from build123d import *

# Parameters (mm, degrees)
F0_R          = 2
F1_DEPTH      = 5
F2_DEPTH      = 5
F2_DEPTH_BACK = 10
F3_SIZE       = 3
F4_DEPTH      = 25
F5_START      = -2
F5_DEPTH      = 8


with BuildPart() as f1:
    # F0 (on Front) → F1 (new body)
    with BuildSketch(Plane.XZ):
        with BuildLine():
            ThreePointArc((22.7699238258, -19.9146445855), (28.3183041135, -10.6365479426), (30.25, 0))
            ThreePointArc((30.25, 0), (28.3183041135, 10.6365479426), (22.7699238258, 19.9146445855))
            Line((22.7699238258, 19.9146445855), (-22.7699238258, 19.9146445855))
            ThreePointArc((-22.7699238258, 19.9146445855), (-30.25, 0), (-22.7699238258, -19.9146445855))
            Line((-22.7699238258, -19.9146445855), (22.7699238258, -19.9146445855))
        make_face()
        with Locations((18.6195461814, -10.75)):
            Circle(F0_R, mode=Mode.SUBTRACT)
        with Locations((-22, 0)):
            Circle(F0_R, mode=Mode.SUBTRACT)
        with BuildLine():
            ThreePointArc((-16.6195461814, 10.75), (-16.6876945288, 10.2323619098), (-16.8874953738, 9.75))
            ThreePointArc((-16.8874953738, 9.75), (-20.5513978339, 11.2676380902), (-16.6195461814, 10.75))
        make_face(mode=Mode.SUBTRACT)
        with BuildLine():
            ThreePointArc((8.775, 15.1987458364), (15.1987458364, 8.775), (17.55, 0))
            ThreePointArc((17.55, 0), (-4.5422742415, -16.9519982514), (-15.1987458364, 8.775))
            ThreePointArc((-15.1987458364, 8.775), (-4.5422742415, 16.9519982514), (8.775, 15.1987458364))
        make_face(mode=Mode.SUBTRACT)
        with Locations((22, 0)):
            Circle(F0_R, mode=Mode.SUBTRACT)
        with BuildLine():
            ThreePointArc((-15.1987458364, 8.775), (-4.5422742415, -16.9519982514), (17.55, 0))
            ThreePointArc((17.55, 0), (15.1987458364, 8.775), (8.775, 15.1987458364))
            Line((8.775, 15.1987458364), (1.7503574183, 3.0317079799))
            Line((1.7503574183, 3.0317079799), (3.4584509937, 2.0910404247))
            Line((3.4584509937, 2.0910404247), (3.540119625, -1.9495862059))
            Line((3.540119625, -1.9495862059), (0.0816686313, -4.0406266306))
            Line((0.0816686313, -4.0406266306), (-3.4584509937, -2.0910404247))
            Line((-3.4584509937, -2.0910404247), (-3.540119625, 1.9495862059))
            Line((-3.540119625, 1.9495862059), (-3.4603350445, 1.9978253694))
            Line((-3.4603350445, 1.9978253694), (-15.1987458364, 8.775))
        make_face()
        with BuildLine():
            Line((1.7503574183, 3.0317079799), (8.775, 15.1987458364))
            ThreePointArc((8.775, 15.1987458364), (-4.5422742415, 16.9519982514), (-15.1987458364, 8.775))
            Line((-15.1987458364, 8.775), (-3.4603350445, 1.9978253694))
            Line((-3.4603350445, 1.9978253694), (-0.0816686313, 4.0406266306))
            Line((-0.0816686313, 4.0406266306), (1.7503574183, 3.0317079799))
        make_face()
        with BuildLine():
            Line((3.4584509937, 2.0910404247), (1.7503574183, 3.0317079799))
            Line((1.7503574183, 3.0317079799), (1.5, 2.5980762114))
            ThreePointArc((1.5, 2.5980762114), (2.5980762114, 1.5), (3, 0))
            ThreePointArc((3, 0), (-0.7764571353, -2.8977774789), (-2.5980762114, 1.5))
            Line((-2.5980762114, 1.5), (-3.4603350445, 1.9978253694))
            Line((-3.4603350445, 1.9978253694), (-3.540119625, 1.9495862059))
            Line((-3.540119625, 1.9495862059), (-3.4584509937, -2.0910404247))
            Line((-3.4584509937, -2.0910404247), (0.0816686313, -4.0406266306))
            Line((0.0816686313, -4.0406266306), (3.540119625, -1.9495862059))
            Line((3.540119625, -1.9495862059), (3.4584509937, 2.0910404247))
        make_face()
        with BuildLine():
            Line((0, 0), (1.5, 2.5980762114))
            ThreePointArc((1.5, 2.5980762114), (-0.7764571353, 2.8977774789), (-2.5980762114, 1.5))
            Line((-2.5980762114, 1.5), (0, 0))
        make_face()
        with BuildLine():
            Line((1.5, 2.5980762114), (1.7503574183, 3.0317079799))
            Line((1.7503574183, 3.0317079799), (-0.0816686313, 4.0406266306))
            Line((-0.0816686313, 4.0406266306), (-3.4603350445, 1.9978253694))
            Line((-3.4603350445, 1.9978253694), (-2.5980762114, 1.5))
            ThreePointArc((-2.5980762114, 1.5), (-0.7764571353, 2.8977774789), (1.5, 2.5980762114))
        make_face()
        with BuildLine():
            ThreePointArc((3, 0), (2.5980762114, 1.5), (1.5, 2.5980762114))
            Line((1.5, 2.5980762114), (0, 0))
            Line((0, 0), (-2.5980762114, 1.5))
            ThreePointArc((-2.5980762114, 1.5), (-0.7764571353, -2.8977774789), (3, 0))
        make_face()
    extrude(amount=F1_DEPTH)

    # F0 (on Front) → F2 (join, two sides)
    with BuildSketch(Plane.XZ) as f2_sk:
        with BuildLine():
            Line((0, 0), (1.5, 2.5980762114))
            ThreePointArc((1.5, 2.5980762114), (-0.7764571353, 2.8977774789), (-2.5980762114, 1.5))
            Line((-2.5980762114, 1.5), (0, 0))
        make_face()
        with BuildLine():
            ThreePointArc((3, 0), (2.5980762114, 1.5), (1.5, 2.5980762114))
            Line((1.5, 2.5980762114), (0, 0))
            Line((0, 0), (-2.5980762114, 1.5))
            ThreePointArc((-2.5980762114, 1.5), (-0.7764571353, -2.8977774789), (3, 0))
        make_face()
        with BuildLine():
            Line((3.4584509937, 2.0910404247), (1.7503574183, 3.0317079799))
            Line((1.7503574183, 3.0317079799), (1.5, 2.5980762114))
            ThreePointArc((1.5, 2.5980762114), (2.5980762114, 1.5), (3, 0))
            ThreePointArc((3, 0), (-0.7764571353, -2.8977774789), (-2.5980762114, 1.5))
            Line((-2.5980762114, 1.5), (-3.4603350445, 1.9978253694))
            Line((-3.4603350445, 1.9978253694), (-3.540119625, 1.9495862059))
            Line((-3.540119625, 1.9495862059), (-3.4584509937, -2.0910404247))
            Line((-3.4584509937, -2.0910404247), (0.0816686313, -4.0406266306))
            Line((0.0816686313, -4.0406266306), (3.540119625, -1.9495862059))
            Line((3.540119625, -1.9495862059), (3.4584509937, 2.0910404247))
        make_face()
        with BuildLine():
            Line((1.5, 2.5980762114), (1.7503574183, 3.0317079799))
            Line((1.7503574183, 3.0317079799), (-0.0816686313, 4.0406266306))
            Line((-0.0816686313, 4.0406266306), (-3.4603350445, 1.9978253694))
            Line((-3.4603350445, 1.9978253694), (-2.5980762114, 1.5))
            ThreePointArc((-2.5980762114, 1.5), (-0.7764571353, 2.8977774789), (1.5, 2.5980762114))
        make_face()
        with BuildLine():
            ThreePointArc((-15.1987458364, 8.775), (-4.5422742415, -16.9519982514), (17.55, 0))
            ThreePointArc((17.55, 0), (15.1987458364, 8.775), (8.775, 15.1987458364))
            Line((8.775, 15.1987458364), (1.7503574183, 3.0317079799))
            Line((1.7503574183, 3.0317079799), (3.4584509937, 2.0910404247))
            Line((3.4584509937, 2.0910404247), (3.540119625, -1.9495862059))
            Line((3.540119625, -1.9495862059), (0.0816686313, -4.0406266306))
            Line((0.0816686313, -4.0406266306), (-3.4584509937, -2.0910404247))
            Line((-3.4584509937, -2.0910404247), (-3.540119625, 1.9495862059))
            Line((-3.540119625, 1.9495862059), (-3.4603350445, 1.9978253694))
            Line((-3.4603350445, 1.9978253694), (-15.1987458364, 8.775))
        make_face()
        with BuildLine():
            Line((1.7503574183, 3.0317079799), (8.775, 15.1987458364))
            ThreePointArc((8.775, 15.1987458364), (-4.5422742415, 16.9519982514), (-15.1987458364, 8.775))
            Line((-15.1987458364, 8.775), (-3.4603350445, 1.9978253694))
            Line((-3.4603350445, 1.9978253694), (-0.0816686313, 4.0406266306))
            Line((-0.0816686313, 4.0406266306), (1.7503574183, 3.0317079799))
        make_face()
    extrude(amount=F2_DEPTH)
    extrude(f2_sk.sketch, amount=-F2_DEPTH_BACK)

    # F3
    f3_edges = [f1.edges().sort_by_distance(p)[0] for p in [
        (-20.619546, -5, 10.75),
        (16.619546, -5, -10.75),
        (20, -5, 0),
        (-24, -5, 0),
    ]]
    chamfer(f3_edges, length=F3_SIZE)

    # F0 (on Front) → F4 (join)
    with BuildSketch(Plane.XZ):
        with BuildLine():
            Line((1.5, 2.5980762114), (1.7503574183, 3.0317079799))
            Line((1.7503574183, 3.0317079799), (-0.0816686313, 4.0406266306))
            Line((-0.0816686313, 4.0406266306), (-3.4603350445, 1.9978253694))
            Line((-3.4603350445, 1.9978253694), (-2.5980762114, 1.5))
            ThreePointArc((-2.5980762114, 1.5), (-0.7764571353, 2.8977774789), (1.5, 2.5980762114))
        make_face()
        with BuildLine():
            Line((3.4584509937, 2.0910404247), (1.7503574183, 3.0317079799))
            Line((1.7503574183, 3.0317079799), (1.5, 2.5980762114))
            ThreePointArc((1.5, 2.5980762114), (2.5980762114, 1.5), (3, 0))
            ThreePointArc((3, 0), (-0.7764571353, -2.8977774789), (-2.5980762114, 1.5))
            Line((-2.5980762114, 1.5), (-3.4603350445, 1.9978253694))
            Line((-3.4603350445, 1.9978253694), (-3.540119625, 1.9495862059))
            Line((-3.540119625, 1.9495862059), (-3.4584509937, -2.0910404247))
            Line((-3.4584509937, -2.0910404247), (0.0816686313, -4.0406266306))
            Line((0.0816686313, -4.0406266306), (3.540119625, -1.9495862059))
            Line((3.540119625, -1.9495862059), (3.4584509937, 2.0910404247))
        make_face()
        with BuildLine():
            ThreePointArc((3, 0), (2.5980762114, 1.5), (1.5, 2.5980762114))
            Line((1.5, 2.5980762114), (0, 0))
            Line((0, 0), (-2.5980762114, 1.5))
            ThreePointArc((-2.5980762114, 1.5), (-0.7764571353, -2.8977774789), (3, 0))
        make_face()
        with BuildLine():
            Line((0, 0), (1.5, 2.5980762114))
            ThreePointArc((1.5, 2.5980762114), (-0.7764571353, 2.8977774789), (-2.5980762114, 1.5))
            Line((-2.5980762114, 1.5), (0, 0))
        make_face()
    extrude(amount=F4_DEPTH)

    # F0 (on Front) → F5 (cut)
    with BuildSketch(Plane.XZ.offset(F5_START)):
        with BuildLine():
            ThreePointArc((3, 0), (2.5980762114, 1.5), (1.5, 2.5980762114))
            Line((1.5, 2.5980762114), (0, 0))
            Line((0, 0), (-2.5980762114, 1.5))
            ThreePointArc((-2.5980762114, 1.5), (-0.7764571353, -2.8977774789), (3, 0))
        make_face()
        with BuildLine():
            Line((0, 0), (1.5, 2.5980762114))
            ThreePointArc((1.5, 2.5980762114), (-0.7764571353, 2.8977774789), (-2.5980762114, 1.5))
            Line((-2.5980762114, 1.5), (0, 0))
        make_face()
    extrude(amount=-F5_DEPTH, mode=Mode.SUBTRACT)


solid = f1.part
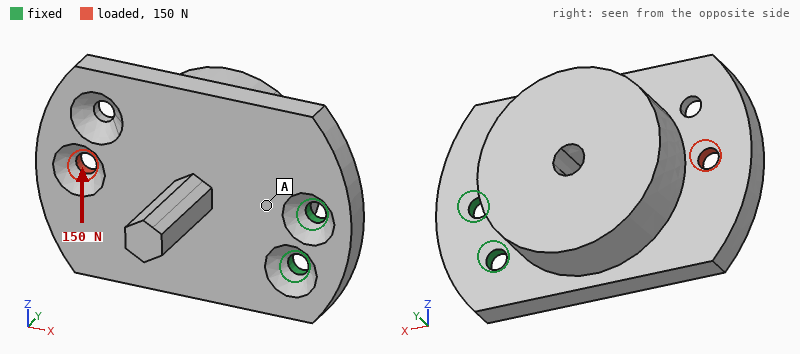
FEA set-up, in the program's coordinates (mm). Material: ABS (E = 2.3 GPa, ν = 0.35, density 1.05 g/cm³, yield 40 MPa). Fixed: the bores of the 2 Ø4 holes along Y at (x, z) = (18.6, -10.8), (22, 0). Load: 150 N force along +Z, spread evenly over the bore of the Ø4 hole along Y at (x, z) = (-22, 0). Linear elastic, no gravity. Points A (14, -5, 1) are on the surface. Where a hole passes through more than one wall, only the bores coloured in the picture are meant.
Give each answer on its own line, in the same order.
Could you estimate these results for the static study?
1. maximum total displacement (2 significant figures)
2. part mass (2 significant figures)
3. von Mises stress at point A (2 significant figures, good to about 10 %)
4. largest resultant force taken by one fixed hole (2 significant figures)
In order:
0.38 mm
22 g
4.1 MPa
480 N
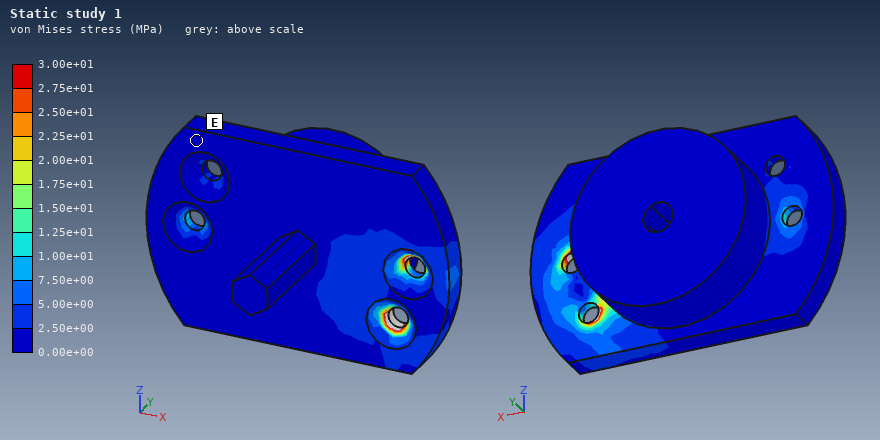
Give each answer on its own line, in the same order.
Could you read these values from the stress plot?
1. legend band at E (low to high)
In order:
0.00e+00 to 2.50e+00 MPa
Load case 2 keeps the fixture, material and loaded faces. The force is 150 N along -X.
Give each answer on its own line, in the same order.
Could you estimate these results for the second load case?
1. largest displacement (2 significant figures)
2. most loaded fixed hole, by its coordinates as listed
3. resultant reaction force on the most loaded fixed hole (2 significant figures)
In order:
94 µm
(22, 0)
130 N
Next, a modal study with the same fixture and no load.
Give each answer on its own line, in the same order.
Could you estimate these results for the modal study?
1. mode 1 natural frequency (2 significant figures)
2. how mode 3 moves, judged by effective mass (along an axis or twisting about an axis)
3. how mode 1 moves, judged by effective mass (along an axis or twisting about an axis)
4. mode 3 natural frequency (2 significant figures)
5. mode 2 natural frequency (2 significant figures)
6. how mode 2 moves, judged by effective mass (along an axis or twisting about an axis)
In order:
330 Hz
twisting about X
along Y
1400 Hz
1200 Hz
along Z
